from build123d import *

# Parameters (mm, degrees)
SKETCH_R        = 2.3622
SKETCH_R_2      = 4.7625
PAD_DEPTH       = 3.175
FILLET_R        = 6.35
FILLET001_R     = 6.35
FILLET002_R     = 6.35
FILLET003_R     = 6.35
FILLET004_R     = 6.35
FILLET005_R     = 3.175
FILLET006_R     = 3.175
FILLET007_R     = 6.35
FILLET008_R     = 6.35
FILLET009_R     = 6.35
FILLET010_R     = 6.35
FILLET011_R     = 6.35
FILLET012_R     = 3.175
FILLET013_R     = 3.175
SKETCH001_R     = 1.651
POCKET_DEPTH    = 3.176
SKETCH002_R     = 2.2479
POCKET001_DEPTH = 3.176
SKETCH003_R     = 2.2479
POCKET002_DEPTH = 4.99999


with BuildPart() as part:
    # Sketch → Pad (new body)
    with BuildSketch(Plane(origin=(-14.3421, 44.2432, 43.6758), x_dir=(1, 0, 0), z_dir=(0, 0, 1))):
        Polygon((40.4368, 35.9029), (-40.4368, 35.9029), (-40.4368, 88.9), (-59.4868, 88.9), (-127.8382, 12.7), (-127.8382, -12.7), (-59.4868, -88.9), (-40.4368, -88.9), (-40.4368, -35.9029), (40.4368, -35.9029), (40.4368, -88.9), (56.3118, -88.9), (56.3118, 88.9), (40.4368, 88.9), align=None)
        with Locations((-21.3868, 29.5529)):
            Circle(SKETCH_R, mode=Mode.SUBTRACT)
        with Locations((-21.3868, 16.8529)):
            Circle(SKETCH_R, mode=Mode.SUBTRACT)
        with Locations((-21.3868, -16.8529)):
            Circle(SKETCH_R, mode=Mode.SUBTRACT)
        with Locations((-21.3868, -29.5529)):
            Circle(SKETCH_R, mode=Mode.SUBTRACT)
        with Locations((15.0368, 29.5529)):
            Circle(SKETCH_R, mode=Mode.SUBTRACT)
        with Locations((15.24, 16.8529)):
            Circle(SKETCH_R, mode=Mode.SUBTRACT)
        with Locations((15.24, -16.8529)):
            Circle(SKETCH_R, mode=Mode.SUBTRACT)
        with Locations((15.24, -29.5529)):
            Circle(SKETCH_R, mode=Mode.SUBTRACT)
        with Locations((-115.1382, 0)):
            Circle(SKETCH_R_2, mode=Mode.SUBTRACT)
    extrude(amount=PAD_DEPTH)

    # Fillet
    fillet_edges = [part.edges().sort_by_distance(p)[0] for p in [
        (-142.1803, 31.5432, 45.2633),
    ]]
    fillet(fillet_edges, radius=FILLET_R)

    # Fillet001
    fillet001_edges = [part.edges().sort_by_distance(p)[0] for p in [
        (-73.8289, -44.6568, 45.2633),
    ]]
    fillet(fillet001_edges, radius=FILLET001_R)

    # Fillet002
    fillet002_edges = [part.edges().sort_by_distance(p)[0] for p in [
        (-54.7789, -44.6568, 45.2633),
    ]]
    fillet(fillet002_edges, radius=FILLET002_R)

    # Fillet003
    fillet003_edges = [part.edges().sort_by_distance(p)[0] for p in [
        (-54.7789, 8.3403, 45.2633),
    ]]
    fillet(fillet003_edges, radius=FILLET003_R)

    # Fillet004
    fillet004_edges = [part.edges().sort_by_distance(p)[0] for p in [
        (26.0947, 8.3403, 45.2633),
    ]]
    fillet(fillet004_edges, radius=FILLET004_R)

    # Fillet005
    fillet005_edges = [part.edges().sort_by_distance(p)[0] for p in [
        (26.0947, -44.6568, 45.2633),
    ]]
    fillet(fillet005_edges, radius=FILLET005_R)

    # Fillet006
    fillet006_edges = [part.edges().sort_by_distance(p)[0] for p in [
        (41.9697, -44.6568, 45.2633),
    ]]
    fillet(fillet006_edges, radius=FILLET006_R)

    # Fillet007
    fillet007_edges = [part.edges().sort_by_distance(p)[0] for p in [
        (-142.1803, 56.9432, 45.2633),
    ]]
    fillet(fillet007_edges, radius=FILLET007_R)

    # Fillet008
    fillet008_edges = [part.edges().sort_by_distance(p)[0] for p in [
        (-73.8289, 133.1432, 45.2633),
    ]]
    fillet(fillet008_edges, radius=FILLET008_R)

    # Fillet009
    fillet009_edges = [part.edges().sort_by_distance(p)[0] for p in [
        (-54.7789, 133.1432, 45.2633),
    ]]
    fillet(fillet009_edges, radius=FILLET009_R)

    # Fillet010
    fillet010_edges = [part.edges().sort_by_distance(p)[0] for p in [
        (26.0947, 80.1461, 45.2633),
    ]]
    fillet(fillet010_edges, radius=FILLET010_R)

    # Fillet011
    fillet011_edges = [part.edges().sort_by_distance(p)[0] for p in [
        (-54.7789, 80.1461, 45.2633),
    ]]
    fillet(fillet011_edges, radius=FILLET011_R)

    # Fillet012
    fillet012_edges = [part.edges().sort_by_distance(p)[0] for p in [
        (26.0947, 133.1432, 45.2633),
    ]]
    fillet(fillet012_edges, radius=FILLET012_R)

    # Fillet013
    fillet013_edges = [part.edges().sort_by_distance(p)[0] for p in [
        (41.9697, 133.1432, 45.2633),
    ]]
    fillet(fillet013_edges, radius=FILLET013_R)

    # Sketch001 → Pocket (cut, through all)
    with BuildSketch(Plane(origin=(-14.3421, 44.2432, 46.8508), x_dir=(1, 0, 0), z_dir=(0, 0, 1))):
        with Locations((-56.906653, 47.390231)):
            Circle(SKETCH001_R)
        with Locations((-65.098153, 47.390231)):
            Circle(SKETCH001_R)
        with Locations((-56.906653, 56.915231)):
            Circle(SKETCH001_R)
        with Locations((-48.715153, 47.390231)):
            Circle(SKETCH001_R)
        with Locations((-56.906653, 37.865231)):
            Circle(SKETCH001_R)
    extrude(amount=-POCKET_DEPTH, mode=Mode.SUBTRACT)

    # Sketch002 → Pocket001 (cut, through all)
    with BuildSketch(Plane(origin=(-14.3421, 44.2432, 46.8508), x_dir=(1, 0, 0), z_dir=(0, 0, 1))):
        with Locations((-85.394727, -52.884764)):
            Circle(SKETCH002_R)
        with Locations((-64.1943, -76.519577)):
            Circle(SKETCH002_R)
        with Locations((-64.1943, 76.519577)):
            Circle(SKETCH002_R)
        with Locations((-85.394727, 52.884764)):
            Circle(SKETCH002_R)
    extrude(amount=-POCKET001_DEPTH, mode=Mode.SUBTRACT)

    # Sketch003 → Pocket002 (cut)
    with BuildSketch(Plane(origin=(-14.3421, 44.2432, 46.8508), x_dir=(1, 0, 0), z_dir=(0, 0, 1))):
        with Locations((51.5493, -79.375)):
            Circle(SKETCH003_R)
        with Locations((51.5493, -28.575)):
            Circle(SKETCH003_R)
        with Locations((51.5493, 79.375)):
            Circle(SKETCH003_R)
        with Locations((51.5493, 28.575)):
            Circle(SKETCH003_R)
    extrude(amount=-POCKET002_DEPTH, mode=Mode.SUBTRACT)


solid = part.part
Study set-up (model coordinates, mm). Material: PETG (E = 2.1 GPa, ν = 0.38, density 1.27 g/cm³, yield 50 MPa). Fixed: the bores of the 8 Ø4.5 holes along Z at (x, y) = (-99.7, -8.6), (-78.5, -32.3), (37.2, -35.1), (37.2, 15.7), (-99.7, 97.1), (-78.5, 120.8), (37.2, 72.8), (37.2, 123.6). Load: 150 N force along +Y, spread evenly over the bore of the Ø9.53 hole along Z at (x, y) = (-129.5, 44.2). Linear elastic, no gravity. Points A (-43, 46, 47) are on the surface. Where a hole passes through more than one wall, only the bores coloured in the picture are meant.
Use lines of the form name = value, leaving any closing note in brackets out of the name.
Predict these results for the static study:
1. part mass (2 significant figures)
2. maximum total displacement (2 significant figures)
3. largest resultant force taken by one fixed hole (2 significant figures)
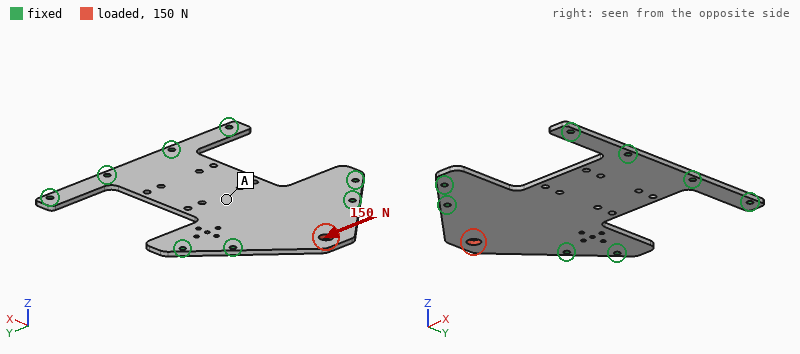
part mass = 75 g
maximum total displacement = 50 µm
largest resultant force taken by one fixed hole = 73 N
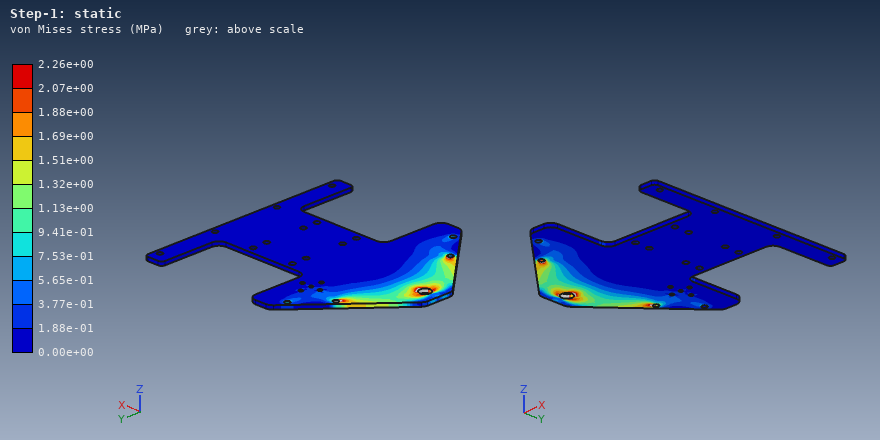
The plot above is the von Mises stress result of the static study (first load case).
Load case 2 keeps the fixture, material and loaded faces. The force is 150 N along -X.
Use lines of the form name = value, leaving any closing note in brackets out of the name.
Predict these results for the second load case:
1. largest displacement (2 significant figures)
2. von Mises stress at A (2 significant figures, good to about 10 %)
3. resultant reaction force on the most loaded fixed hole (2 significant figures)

largest displacement = 47 µm
von Mises stress at A = 0.35 MPa
resultant reaction force on the most loaded fixed hole = 50 N
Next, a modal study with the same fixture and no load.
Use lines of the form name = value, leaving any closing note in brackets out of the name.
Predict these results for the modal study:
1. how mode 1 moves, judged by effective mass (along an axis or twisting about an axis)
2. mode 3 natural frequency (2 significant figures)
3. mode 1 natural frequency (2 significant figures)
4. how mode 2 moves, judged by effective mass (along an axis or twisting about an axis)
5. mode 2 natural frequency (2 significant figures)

how mode 1 moves, judged by effective mass = along Z
mode 3 natural frequency = 420 Hz
mode 1 natural frequency = 210 Hz
how mode 2 moves, judged by effective mass = along Z
mode 2 natural frequency = 250 Hz
